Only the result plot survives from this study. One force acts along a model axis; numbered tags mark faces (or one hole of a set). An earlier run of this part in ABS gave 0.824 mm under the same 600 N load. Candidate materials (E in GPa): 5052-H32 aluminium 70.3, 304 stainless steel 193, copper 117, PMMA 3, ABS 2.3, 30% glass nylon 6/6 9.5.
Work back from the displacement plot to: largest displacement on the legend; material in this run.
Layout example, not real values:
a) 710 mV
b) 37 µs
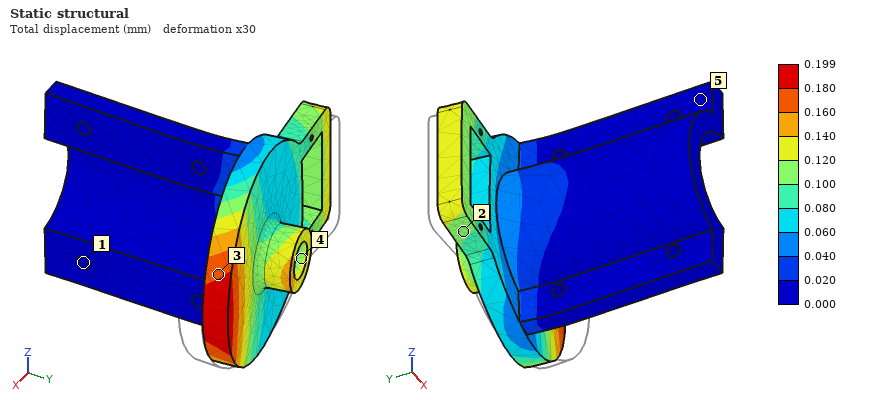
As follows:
a) 0.199 mm
b) 30% glass nylon 6/6
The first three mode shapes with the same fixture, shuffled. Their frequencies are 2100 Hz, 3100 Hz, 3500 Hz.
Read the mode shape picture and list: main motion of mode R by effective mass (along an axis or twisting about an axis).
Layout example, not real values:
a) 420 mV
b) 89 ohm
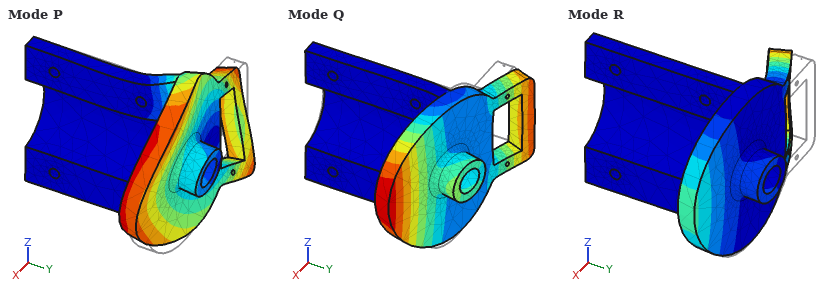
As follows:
a) along Y
